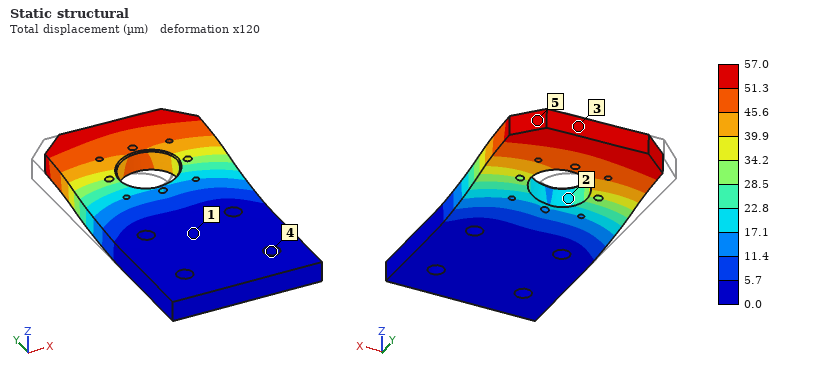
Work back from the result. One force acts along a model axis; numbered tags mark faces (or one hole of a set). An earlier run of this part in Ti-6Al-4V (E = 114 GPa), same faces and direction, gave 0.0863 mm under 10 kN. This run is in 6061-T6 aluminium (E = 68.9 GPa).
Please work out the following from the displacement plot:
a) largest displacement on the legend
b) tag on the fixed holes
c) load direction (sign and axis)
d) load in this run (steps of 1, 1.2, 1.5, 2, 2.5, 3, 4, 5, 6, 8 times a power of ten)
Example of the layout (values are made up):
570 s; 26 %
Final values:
57.0 µm; 4; +X; 4 kN
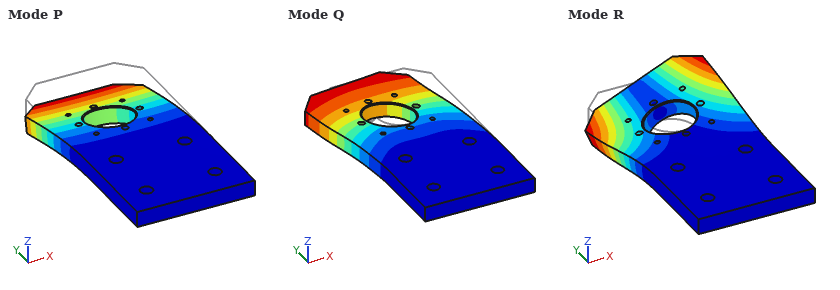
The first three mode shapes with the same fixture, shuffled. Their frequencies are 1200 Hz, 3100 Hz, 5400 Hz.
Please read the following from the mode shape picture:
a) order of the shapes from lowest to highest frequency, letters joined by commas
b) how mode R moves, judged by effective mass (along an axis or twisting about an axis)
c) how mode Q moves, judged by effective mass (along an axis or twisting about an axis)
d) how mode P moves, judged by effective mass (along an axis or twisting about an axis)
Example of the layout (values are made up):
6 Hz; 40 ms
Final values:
P, R, Q; twisting about Y; along X; along Z
